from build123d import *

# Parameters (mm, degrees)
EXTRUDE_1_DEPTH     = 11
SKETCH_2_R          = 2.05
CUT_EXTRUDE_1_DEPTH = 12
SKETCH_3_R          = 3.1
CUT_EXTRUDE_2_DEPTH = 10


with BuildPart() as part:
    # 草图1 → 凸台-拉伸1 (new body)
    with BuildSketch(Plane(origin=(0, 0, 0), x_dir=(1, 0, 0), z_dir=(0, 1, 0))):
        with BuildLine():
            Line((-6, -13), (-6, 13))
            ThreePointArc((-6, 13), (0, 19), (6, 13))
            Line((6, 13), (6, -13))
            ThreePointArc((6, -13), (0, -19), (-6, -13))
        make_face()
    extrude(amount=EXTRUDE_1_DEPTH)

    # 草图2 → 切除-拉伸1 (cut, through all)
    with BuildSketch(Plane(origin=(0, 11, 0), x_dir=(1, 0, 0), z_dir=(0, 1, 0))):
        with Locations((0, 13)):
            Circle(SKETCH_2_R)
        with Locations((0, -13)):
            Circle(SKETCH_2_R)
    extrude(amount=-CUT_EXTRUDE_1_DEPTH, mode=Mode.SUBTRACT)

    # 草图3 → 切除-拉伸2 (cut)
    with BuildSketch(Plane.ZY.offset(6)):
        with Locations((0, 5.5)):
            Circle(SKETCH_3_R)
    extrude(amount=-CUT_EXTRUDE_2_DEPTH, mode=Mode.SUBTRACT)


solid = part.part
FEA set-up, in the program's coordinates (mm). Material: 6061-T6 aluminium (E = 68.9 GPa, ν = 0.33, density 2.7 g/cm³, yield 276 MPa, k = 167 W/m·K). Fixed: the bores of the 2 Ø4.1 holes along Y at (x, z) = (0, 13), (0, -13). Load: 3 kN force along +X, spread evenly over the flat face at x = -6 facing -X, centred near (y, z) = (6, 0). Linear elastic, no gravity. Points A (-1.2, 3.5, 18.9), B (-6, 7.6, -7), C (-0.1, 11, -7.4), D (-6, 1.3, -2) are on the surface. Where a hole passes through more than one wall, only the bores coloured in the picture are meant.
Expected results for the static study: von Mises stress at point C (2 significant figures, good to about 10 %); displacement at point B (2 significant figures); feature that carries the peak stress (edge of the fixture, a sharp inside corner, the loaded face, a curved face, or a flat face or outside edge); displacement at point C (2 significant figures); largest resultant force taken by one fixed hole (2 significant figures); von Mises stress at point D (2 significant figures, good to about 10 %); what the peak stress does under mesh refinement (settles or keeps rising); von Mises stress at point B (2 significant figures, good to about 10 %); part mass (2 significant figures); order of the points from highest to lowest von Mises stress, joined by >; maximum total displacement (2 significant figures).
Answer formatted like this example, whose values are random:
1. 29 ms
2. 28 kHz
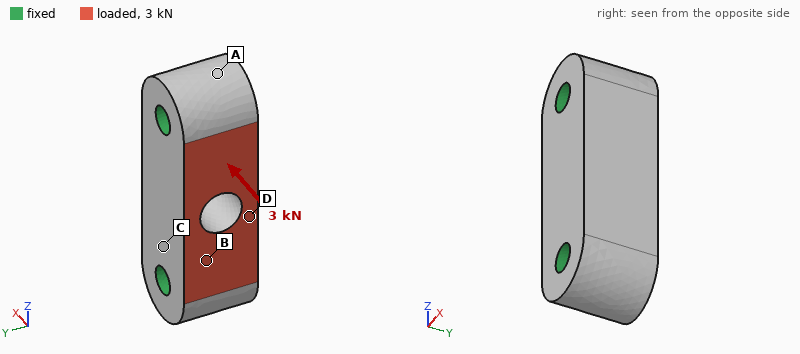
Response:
1. 17 MPa
2. 4.3 µm
3. edge of the fixture
4. 2.9 µm
5. 1.5 kN
6. 27 MPa
7. keeps rising
8. 9.7 MPa
9. 11 g
10. D > C > B > A
11. 6.2 µm
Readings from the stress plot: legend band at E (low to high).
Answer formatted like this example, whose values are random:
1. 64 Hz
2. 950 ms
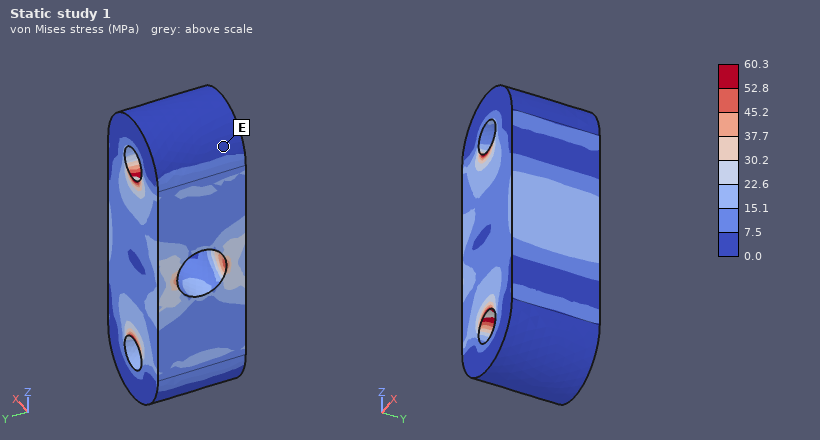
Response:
1. 0.0 to 7.5 MPa
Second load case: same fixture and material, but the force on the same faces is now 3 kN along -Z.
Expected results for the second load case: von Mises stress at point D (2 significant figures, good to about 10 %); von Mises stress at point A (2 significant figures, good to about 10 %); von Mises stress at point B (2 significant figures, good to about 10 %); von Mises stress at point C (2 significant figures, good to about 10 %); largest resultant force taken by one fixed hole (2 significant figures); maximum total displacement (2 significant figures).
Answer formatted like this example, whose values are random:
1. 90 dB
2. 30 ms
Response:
1. 22 MPa
2. 4.8 MPa
3. 22 MPa
4. 9.4 MPa
5. 1.6 kN
6. 3.8 µm
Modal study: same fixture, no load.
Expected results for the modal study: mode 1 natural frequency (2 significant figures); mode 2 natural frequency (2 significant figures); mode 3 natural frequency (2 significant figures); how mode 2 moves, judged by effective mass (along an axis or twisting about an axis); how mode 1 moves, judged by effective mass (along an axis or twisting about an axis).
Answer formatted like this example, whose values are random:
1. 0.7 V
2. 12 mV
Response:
1. 46 kHz
2. 53 kHz
3. 59 kHz
4. along Y
5. along X
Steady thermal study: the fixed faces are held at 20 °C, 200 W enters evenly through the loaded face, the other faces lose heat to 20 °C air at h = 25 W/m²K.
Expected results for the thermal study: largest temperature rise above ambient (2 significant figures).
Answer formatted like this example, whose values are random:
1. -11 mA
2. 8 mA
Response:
1. 45 K
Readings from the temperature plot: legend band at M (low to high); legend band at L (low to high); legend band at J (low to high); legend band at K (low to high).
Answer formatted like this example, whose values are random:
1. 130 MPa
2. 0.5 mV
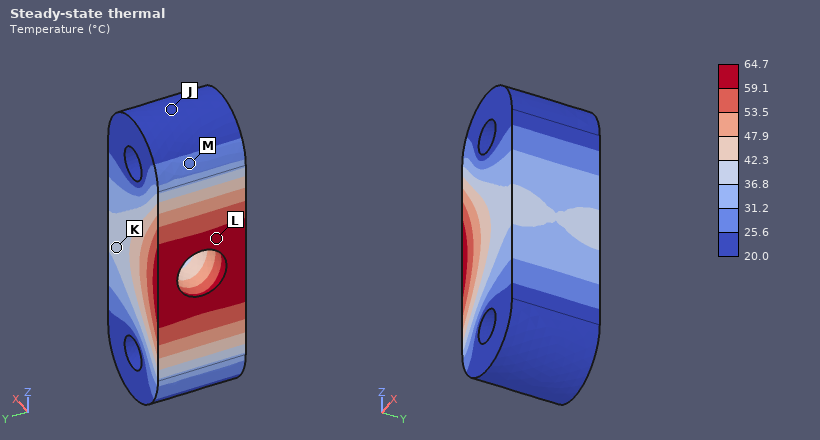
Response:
1. 25.6 to 31.2 °C
2. 59.1 to 64.7 °C
3. 20.0 to 25.6 °C
4. 36.8 to 42.3 °C
